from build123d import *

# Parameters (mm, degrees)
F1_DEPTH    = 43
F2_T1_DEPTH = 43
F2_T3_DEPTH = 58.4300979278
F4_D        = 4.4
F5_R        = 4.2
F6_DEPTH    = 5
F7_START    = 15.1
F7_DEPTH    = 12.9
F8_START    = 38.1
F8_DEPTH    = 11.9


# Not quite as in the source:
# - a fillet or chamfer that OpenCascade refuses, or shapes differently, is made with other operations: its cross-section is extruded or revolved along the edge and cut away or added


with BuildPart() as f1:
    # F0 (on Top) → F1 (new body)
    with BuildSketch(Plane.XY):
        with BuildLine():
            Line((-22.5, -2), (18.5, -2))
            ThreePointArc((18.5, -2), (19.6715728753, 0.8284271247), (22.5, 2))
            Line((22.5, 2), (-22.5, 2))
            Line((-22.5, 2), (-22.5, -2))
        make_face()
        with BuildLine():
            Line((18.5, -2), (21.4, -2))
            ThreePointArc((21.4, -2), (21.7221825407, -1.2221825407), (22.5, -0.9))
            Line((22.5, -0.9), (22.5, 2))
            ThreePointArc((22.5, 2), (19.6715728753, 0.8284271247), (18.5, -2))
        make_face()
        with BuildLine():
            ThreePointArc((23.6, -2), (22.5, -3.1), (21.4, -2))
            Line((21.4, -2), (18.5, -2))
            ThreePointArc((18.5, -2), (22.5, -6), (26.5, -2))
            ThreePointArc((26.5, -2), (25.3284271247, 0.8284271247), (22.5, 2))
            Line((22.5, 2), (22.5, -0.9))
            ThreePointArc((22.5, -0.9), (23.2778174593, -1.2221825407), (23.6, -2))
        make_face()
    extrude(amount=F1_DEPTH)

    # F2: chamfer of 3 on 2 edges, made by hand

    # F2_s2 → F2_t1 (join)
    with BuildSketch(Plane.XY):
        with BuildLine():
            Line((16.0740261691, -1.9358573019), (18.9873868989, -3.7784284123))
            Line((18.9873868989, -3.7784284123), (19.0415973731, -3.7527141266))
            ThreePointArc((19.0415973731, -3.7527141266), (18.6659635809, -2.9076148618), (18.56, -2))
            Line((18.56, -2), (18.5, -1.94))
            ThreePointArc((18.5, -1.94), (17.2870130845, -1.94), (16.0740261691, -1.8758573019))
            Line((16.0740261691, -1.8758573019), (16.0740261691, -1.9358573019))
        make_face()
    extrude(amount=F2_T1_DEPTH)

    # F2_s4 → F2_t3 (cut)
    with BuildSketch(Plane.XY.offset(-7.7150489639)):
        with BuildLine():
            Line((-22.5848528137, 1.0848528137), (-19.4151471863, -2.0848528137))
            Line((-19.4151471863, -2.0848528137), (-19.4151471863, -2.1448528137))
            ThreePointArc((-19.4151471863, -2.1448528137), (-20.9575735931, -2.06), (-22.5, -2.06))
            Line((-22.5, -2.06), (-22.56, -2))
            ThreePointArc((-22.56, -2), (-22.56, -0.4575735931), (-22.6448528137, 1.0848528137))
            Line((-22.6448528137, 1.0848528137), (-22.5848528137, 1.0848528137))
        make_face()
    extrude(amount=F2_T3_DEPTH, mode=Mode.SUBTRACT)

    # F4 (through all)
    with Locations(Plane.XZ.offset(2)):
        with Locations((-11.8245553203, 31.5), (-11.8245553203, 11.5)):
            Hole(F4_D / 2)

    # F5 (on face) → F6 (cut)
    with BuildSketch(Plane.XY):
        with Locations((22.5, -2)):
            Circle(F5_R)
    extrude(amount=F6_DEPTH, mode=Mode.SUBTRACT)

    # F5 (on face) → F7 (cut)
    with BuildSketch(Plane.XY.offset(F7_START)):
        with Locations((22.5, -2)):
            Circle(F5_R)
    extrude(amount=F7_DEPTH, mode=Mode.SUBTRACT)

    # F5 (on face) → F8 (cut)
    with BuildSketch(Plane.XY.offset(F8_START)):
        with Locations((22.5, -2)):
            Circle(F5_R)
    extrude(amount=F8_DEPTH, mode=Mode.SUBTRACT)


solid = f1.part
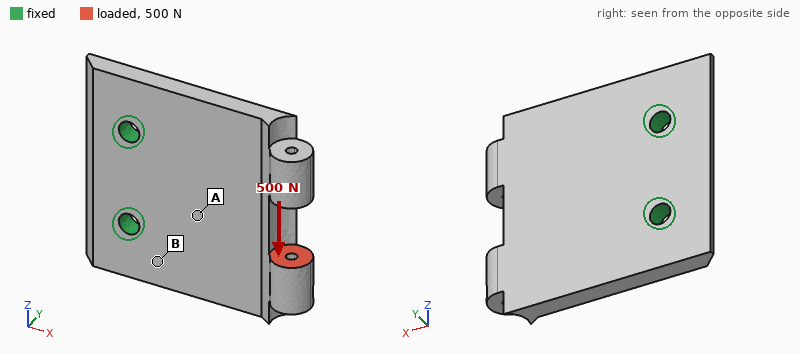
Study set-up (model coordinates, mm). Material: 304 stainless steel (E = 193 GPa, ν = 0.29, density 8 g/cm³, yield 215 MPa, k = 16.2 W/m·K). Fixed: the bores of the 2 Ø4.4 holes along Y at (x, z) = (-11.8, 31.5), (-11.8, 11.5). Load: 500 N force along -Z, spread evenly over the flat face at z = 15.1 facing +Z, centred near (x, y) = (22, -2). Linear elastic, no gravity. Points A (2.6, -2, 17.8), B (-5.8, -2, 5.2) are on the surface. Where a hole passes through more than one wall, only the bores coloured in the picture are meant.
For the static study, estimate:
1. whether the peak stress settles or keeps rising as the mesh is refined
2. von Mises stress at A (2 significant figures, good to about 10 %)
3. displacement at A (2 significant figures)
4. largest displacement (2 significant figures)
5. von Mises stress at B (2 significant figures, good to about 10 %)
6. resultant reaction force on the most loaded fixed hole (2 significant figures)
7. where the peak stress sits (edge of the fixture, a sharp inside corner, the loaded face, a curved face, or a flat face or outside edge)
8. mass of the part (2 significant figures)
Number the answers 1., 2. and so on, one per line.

1. keeps rising
2. 16 MPa
3. 1.7 µm
4. 11 µm
5. 6.0 MPa
6. 790 N
7. a sharp inside corner
8. 63 g
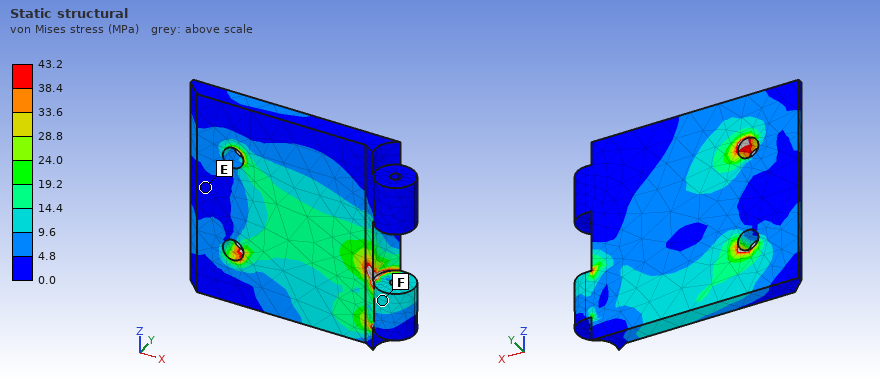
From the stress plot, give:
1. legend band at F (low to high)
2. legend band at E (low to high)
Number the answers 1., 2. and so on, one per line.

1. 9.6 to 14.4 MPa
2. 0.0 to 4.8 MPa
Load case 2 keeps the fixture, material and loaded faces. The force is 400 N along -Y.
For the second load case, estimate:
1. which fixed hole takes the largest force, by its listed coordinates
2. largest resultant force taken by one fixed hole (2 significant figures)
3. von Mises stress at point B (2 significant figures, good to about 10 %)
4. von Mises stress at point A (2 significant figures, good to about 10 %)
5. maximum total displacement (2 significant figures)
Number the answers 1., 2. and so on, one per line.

1. (-11.8, 11.5)
2. 300 N
3. 98 MPa
4. 74 MPa
5. 0.17 mm
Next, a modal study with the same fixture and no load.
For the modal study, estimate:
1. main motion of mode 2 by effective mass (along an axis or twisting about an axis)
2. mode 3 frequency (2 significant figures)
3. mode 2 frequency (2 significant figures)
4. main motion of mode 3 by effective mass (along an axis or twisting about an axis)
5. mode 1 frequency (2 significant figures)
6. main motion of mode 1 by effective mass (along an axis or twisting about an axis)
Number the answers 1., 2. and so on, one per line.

1. twisting about X
2. 12 kHz
3. 4500 Hz
4. along Z
5. 2300 Hz
6. along Y
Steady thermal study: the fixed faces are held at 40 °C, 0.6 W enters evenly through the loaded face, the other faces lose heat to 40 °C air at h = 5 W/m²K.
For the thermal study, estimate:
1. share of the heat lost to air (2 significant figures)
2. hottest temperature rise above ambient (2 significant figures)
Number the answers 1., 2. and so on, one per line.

1. 13 %
2. 14 K
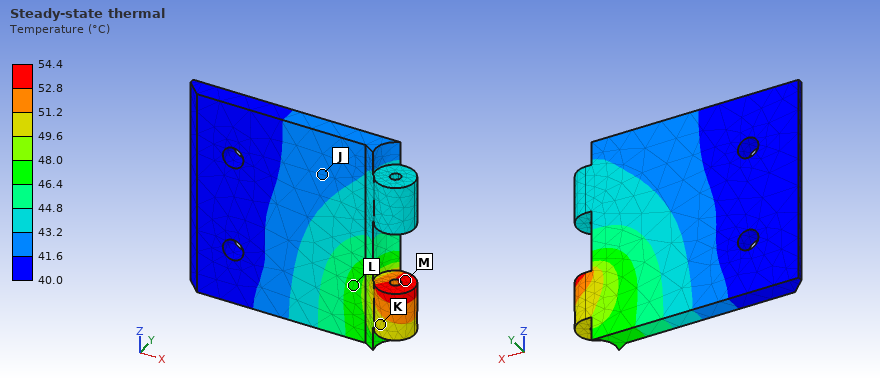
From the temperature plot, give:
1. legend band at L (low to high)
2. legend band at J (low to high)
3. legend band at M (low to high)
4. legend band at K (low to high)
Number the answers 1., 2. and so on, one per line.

1. 46.4 to 48.0 °C
2. 41.6 to 43.2 °C
3. 52.8 to 54.4 °C
4. 49.6 to 51.2 °C
